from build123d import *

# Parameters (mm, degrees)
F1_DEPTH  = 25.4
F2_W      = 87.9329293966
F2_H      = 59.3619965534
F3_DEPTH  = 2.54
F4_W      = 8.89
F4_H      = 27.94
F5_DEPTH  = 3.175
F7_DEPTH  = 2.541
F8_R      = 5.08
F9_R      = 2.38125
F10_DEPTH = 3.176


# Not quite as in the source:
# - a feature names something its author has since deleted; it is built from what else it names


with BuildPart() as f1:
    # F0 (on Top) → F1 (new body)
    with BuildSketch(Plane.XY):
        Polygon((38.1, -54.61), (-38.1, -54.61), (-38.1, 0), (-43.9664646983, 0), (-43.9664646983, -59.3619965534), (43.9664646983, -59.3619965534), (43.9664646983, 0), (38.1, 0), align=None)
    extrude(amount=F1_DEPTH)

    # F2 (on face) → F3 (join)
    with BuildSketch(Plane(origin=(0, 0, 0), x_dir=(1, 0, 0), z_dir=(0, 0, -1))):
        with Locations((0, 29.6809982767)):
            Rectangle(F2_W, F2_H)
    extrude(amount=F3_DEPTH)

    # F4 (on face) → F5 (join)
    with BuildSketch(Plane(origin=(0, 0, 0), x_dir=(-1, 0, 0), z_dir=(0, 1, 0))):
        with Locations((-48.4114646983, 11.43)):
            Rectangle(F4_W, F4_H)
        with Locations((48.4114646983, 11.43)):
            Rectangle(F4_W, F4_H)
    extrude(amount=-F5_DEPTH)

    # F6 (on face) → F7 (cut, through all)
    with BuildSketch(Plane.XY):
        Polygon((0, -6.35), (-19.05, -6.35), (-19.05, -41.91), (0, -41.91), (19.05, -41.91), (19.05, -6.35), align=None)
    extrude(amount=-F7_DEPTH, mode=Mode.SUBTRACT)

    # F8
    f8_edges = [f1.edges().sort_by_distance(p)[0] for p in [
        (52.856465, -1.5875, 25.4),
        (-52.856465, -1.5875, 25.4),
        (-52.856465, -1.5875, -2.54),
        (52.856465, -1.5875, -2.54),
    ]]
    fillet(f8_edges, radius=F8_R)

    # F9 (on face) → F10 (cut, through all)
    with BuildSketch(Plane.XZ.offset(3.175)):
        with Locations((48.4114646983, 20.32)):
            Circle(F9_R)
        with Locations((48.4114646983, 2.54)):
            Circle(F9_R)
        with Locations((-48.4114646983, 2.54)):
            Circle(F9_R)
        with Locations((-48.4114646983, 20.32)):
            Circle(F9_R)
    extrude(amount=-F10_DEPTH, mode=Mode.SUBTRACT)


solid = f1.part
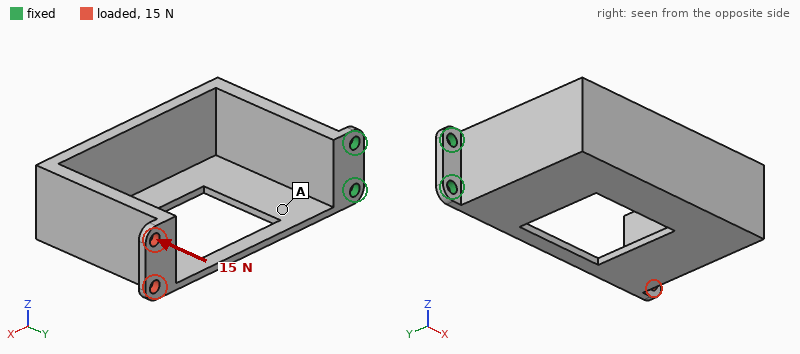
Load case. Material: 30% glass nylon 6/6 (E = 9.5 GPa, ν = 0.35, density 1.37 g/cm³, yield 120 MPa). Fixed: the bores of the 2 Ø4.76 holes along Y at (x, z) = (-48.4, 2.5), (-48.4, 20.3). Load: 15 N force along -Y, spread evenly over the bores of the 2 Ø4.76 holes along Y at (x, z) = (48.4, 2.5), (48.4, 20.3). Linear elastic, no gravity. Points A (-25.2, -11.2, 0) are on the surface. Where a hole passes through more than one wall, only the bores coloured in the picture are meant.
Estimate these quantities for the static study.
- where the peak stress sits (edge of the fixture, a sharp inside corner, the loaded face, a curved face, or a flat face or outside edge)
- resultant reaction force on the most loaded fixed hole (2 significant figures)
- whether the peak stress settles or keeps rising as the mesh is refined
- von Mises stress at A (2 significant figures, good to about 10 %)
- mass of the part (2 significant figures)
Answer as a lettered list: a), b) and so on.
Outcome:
a) edge of the fixture
b) 19 N
c) keeps rising
d) 2.3 MPa
e) 52 g
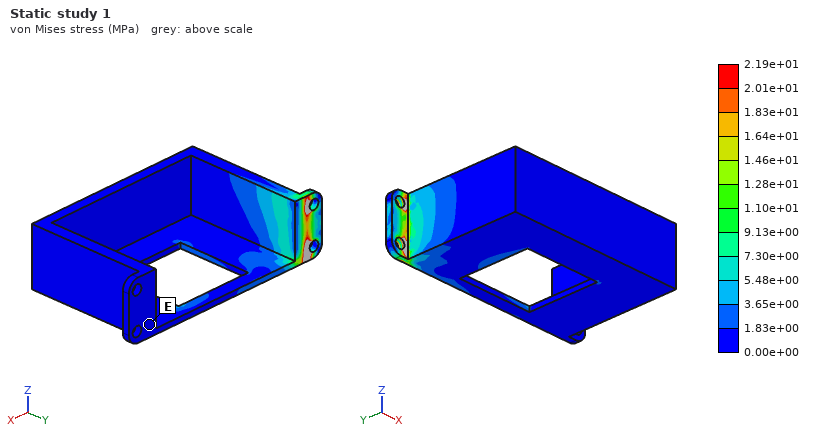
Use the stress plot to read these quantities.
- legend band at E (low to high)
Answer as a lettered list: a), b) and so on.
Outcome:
a) 0.00e+00 to 1.83e+00 MPa
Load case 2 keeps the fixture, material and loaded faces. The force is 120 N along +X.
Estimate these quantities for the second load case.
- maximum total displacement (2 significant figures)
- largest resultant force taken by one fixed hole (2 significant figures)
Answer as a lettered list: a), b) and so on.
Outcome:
a) 1.5 mm
b) 61 N
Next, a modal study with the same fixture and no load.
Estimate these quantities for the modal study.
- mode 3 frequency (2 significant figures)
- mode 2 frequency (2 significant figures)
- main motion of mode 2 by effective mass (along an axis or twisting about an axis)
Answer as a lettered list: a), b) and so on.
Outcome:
a) 390 Hz
b) 140 Hz
c) along Z
